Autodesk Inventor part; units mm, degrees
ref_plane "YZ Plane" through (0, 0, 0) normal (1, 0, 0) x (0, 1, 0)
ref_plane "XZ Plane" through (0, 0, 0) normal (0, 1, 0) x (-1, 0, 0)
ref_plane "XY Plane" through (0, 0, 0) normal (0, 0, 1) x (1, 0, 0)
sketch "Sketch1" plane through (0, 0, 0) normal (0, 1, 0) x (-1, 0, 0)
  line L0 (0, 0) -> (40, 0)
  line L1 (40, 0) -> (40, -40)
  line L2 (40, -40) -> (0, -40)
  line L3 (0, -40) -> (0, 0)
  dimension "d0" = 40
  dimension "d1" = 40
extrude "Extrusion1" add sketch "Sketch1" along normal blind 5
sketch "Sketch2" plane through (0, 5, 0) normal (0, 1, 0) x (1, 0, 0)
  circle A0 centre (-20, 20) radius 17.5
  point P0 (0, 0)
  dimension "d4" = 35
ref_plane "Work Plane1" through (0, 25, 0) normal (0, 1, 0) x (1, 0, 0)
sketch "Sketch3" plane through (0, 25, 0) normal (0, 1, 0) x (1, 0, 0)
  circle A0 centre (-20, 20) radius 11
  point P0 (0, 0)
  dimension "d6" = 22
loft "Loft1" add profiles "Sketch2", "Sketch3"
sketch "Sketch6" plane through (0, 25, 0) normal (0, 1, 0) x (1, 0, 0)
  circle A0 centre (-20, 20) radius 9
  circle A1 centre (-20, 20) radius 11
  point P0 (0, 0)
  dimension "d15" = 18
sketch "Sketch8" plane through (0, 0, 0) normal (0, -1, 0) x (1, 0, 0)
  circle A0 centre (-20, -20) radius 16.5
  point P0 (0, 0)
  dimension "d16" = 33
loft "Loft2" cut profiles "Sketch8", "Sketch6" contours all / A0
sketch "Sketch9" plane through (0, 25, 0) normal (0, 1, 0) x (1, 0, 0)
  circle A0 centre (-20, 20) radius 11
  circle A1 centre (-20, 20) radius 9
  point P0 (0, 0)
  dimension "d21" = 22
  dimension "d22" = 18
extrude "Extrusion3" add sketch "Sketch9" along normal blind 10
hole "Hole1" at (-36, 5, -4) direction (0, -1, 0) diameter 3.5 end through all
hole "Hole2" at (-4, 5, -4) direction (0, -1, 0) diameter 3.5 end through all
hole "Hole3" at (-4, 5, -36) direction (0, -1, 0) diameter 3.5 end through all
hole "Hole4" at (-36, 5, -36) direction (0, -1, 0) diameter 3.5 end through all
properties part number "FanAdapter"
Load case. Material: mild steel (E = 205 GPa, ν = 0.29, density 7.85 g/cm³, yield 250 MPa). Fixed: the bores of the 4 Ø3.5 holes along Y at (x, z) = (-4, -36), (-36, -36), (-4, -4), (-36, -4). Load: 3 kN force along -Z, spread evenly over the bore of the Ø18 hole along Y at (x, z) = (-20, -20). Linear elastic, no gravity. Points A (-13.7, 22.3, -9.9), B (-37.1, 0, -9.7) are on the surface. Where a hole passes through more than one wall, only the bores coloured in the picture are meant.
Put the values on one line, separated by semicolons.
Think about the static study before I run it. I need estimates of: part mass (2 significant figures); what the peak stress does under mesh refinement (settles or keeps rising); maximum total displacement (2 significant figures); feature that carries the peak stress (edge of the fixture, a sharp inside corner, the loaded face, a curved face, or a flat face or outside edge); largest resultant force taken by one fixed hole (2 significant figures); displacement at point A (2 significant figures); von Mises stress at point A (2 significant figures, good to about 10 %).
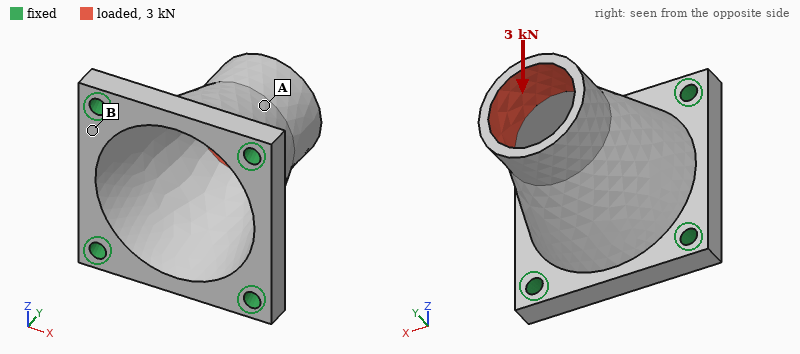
70 g; keeps rising; 28 µm; edge of the fixture; 1.7 kN; 16 µm; 44 MPa
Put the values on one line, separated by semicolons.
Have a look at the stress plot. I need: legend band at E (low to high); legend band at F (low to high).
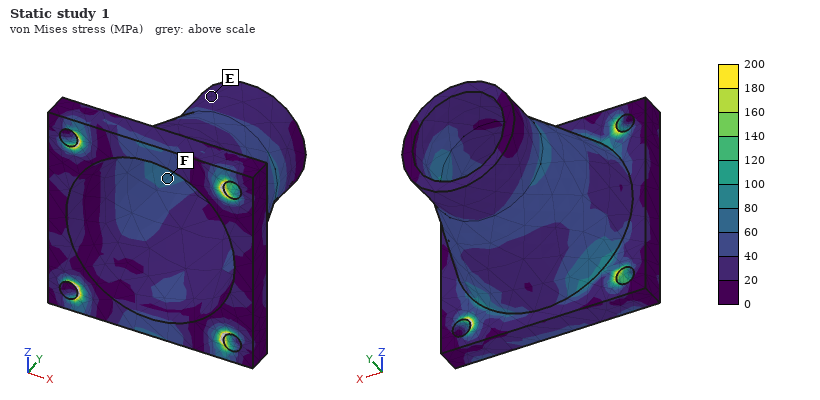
20 to 40 MPa; 60 to 80 MPa
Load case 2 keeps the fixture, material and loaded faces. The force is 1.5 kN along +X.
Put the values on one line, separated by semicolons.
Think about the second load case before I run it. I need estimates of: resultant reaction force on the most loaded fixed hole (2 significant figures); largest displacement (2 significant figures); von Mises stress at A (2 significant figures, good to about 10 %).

840 N; 14 µm; 26 MPa
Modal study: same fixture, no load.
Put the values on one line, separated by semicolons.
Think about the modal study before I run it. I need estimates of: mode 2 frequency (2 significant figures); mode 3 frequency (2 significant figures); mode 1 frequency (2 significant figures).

14 kHz; 14 kHz; 14 kHz
